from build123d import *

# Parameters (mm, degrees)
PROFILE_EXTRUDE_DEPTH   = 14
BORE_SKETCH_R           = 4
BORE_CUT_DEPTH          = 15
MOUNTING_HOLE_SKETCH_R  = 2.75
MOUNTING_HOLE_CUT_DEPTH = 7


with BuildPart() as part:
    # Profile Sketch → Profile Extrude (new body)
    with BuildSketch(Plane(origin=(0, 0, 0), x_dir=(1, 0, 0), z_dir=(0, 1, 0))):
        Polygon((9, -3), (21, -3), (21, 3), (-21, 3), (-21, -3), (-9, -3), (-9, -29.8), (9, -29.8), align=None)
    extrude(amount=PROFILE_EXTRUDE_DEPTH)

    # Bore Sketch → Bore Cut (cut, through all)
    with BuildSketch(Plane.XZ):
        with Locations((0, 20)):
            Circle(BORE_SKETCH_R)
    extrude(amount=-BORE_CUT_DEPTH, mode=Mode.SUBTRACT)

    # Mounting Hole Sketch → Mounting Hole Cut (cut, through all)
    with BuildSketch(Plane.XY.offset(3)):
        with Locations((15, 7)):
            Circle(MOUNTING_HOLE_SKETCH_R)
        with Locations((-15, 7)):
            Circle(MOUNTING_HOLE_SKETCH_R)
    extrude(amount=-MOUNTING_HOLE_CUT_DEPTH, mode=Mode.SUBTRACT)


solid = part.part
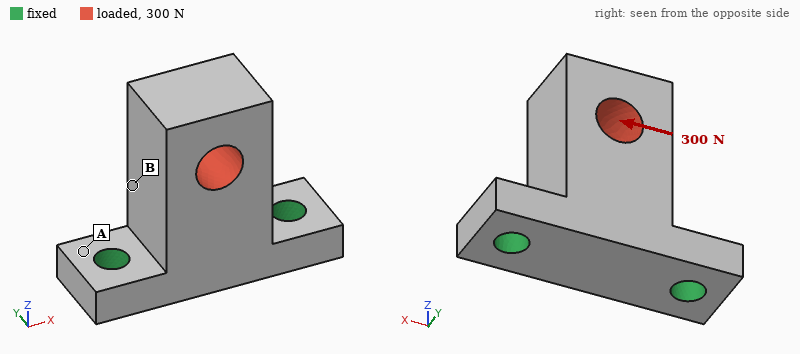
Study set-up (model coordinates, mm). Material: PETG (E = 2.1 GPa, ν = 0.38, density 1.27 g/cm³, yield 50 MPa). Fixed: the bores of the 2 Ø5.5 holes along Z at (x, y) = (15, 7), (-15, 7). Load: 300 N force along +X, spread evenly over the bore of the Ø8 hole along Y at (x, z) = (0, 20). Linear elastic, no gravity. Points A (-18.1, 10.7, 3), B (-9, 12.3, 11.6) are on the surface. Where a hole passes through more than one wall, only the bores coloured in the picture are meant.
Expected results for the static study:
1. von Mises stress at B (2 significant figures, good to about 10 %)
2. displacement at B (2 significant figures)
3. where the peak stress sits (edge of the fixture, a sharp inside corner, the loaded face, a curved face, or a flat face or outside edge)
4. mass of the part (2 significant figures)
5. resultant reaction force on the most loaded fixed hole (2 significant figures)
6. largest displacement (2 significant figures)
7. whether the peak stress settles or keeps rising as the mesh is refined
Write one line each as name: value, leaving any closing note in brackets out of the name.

von Mises stress at B: 4.0 MPa
displacement at B: 0.095 mm
where the peak stress sits: edge of the fixture
mass of the part: 12 g
resultant reaction force on the most loaded fixed hole: 300 N
largest displacement: 0.25 mm
whether the peak stress settles or keeps rising as the mesh is refined: keeps rising
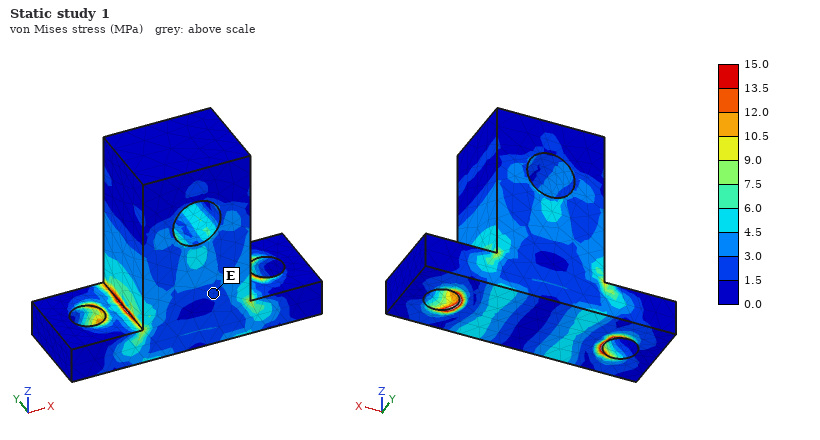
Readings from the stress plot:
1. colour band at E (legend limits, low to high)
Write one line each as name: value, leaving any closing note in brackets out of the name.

colour band at E: 1.5 to 3.0 MPa
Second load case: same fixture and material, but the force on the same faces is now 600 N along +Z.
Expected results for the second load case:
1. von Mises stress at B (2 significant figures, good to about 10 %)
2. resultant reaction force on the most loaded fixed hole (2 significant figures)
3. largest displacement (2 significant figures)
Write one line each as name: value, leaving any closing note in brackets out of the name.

von Mises stress at B: 2.8 MPa
resultant reaction force on the most loaded fixed hole: 320 N
largest displacement: 91 µm
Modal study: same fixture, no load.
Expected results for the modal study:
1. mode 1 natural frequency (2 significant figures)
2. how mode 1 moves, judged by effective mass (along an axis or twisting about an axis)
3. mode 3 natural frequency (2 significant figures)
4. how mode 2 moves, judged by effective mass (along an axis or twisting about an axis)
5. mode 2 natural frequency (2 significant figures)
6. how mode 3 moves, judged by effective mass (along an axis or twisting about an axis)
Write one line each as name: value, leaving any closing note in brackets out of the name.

mode 1 natural frequency: 1300 Hz
how mode 1 moves, judged by effective mass: along Y
mode 3 natural frequency: 4900 Hz
how mode 2 moves, judged by effective mass: along X
mode 2 natural frequency: 2700 Hz
how mode 3 moves, judged by effective mass: along Z
